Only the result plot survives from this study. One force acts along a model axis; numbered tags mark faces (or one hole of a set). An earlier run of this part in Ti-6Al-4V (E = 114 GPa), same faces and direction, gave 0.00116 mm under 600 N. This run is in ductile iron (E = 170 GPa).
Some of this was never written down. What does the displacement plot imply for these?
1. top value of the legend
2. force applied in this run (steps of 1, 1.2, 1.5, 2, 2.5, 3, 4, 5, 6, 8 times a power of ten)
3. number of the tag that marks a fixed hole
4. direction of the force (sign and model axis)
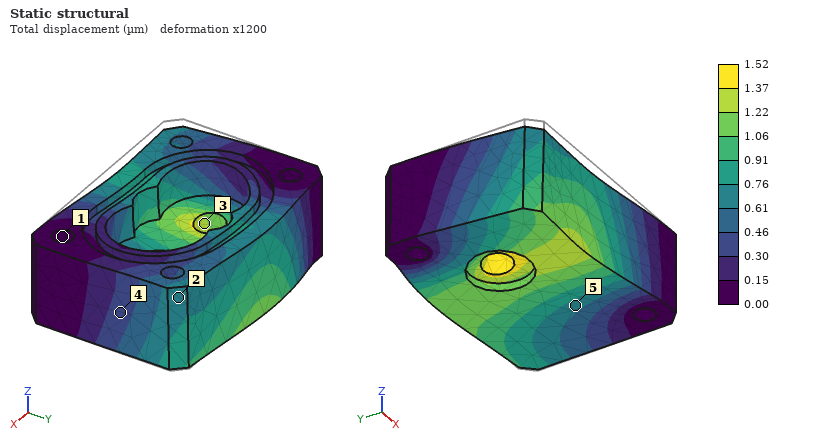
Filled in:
1.52 µm
1.2 kN
1
+Y
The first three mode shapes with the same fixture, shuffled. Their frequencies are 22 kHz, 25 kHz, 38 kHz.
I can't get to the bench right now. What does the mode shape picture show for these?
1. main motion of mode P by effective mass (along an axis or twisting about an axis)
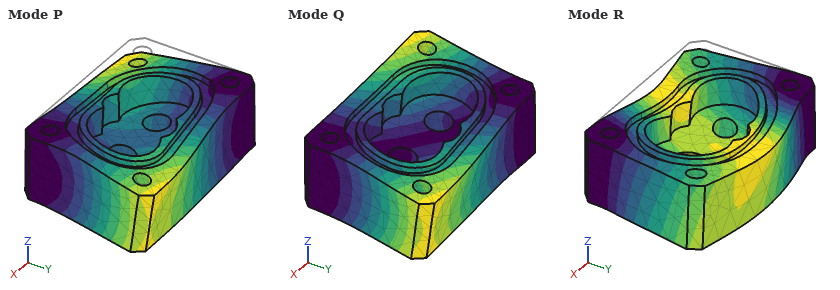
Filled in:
along Z
